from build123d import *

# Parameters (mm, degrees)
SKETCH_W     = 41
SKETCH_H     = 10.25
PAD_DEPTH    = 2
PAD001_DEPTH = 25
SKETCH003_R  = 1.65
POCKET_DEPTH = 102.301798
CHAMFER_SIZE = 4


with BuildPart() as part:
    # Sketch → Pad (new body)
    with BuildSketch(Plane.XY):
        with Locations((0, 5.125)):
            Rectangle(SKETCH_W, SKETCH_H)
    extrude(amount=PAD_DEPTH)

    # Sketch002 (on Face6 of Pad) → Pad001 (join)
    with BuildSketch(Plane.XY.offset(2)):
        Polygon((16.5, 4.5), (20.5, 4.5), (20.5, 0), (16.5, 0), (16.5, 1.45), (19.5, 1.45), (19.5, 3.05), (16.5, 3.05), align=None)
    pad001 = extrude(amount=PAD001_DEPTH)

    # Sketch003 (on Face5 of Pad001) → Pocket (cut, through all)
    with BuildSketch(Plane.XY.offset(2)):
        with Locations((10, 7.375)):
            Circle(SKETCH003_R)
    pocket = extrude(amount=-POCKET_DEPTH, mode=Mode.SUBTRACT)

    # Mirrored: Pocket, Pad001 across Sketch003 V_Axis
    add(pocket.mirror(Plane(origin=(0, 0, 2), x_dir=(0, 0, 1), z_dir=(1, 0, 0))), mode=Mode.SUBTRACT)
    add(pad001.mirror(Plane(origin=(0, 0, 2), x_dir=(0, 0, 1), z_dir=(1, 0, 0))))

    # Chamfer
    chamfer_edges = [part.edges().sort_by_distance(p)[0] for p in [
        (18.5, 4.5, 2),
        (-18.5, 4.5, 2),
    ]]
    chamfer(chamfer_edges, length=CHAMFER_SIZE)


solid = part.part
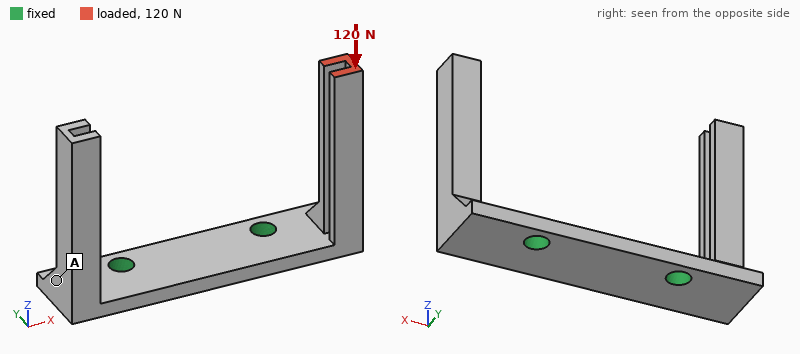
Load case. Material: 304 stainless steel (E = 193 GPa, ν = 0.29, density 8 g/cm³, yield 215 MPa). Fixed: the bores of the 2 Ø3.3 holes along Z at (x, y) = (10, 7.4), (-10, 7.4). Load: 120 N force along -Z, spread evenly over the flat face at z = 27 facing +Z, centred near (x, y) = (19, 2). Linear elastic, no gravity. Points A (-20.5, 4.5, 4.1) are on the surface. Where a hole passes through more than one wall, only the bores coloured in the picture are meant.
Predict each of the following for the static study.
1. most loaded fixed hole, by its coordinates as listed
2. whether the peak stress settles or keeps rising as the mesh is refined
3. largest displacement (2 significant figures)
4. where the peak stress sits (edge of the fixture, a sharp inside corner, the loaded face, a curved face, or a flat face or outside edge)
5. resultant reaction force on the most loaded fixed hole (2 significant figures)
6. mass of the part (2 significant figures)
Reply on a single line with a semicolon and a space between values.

(10, 7.4); keeps rising; 98 µm; edge of the fixture; 130 N; 12 g
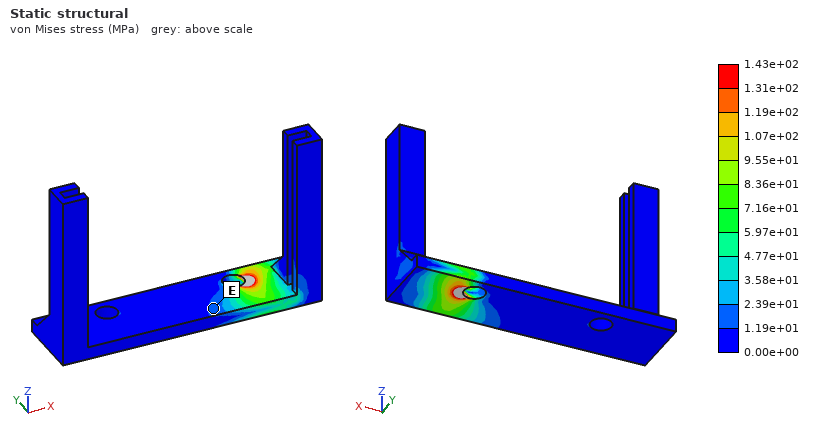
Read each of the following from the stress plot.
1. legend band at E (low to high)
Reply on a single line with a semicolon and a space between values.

1.19e+01 to 2.39e+01 MPa
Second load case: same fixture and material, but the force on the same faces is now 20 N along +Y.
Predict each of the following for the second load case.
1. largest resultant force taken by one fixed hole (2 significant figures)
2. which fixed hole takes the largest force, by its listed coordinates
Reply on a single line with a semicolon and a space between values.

25 N; (10, 7.4)
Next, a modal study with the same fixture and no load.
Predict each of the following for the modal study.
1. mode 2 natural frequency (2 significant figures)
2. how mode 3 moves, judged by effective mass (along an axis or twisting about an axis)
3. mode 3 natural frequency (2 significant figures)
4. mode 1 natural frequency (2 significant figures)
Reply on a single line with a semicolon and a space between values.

2300 Hz; along Y; 3100 Hz; 2300 Hz
